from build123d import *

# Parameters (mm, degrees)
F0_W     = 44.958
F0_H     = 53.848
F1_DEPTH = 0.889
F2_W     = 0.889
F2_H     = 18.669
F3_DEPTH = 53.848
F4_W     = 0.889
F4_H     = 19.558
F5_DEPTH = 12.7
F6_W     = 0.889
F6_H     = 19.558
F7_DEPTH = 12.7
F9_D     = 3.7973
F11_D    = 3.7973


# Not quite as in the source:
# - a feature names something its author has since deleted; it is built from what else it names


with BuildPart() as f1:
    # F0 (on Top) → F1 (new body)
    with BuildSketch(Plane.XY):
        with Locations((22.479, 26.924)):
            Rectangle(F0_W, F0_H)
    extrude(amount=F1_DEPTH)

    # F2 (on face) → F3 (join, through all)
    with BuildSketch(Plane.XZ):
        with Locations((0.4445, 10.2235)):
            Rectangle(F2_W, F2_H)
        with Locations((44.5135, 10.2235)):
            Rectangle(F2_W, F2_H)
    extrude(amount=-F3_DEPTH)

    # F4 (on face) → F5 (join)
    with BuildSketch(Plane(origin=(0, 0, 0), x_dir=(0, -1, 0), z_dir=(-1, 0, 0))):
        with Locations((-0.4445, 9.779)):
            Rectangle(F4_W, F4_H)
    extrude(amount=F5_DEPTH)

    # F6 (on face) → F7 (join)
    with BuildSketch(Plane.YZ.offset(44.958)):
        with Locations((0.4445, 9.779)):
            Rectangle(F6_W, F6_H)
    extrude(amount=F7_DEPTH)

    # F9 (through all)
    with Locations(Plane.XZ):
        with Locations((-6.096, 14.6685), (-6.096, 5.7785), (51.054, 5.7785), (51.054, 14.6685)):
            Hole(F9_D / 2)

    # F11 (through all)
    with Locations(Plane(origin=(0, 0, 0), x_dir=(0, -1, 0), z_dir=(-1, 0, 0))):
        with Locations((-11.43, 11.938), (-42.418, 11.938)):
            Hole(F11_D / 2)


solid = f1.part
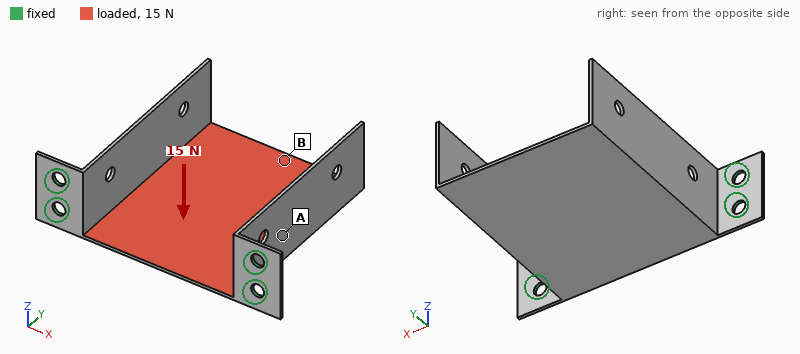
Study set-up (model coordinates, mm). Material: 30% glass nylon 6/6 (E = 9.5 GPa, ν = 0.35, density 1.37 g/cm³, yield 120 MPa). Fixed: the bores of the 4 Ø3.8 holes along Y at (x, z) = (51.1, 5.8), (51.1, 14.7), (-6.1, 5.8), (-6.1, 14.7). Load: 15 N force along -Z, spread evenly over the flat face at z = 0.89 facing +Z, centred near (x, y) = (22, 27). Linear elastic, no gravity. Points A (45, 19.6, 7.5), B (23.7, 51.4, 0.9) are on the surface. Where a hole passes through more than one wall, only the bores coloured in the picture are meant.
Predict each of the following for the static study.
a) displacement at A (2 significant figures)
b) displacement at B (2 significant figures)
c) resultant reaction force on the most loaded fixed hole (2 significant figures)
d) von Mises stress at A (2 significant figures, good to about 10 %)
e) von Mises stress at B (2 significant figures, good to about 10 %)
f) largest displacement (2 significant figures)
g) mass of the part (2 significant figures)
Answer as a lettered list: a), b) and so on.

a) 0.23 mm
b) 0.98 mm
c) 19 N
d) 4.1 MPa
e) 8.1 MPa
f) 1.0 mm
g) 5.9 g
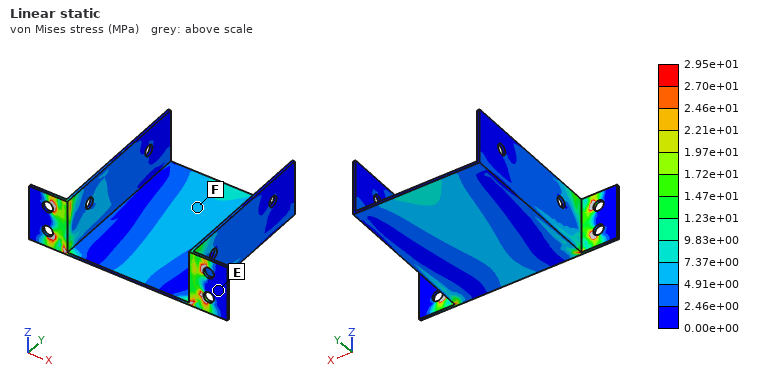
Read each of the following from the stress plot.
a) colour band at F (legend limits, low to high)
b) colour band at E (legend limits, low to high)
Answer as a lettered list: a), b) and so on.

a) 4.91e+00 to 7.37e+00 MPa
b) 0.00e+00 to 2.46e+00 MPa
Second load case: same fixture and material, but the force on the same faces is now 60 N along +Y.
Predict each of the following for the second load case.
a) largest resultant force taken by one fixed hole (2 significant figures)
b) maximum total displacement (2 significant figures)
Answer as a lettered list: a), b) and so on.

a) 43 N
b) 0.81 mm
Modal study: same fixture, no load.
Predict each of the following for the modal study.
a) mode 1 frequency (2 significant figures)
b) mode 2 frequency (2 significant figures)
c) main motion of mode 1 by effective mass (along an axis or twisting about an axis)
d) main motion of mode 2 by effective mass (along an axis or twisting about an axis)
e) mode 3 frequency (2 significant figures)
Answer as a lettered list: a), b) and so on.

a) 370 Hz
b) 430 Hz
c) along Z
d) along X
e) 590 Hz
